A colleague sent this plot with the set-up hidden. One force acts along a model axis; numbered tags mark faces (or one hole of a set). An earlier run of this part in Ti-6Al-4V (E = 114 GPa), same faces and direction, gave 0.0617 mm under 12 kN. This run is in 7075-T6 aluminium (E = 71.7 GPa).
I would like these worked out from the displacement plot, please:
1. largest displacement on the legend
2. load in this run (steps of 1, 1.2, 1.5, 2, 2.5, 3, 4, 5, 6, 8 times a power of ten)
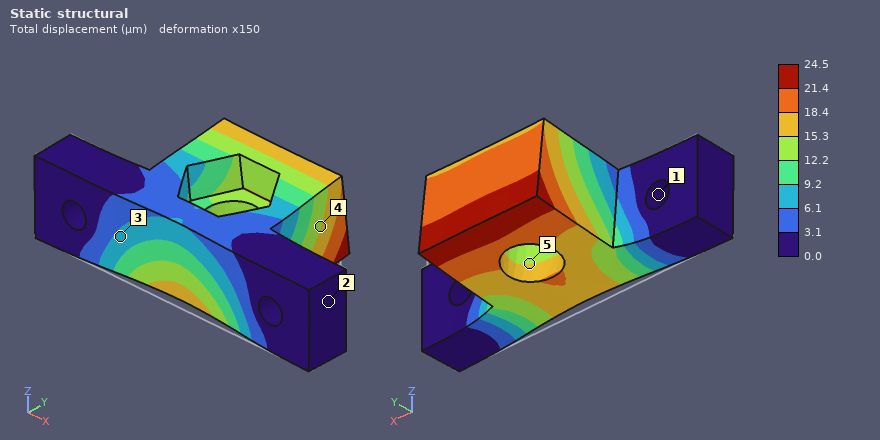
24.5 µm
3 kN
